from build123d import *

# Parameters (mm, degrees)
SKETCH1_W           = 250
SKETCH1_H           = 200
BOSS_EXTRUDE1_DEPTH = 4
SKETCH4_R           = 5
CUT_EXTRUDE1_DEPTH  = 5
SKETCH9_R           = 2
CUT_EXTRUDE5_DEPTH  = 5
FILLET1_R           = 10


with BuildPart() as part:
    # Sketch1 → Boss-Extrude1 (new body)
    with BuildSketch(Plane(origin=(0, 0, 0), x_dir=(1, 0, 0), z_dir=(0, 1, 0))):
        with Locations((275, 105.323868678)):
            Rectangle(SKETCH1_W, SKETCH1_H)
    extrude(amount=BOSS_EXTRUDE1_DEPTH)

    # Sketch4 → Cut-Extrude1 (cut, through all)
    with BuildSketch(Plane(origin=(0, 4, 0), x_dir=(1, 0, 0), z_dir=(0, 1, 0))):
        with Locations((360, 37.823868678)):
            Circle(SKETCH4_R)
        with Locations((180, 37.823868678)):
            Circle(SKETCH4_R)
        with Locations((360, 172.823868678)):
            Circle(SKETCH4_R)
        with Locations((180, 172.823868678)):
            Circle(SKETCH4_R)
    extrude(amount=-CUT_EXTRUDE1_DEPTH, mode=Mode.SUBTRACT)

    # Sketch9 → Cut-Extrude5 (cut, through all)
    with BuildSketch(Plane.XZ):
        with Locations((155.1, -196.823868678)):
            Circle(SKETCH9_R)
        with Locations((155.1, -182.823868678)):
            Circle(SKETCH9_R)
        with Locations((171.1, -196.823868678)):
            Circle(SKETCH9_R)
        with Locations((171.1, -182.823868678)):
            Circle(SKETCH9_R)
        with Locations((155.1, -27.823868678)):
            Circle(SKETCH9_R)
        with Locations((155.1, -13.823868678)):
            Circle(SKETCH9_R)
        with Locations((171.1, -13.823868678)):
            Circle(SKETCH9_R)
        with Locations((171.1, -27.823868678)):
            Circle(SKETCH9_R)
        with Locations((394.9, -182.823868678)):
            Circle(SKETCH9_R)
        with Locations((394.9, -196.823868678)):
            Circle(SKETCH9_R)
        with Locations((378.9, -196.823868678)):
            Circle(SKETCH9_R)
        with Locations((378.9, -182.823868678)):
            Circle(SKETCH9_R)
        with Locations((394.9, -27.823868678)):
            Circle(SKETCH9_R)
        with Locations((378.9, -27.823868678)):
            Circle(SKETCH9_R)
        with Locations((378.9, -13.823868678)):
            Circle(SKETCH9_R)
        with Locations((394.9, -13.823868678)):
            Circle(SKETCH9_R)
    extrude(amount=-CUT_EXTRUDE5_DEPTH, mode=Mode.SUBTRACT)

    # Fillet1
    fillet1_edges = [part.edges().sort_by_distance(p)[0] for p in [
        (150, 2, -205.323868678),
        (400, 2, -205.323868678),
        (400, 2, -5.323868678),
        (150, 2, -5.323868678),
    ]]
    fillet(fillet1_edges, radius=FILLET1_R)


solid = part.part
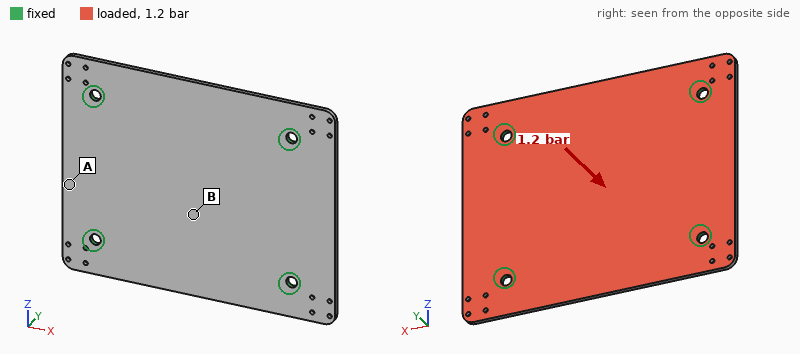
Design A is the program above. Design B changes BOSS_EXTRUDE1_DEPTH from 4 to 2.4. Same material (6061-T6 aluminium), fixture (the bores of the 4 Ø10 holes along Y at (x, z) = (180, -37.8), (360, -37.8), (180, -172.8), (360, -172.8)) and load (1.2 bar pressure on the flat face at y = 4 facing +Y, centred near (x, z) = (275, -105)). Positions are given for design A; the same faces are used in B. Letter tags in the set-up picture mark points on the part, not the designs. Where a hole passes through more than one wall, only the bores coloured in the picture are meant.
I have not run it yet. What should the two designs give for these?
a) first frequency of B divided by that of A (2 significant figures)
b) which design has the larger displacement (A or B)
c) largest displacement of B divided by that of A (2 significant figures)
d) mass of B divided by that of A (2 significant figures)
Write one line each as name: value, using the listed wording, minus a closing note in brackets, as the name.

first frequency of B divided by that of A: 0.61
which design has the larger displacement: B
largest displacement of B divided by that of A: 4.5
mass of B divided by that of A: 0.60
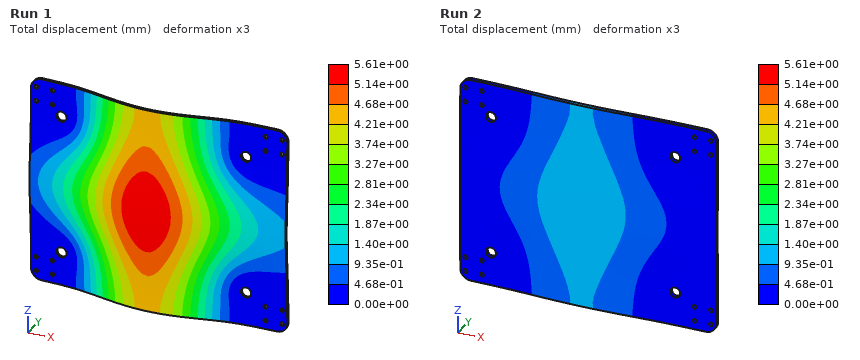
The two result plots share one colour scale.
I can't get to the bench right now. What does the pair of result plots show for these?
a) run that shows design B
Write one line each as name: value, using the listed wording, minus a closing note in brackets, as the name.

run that shows design B: Run 1
